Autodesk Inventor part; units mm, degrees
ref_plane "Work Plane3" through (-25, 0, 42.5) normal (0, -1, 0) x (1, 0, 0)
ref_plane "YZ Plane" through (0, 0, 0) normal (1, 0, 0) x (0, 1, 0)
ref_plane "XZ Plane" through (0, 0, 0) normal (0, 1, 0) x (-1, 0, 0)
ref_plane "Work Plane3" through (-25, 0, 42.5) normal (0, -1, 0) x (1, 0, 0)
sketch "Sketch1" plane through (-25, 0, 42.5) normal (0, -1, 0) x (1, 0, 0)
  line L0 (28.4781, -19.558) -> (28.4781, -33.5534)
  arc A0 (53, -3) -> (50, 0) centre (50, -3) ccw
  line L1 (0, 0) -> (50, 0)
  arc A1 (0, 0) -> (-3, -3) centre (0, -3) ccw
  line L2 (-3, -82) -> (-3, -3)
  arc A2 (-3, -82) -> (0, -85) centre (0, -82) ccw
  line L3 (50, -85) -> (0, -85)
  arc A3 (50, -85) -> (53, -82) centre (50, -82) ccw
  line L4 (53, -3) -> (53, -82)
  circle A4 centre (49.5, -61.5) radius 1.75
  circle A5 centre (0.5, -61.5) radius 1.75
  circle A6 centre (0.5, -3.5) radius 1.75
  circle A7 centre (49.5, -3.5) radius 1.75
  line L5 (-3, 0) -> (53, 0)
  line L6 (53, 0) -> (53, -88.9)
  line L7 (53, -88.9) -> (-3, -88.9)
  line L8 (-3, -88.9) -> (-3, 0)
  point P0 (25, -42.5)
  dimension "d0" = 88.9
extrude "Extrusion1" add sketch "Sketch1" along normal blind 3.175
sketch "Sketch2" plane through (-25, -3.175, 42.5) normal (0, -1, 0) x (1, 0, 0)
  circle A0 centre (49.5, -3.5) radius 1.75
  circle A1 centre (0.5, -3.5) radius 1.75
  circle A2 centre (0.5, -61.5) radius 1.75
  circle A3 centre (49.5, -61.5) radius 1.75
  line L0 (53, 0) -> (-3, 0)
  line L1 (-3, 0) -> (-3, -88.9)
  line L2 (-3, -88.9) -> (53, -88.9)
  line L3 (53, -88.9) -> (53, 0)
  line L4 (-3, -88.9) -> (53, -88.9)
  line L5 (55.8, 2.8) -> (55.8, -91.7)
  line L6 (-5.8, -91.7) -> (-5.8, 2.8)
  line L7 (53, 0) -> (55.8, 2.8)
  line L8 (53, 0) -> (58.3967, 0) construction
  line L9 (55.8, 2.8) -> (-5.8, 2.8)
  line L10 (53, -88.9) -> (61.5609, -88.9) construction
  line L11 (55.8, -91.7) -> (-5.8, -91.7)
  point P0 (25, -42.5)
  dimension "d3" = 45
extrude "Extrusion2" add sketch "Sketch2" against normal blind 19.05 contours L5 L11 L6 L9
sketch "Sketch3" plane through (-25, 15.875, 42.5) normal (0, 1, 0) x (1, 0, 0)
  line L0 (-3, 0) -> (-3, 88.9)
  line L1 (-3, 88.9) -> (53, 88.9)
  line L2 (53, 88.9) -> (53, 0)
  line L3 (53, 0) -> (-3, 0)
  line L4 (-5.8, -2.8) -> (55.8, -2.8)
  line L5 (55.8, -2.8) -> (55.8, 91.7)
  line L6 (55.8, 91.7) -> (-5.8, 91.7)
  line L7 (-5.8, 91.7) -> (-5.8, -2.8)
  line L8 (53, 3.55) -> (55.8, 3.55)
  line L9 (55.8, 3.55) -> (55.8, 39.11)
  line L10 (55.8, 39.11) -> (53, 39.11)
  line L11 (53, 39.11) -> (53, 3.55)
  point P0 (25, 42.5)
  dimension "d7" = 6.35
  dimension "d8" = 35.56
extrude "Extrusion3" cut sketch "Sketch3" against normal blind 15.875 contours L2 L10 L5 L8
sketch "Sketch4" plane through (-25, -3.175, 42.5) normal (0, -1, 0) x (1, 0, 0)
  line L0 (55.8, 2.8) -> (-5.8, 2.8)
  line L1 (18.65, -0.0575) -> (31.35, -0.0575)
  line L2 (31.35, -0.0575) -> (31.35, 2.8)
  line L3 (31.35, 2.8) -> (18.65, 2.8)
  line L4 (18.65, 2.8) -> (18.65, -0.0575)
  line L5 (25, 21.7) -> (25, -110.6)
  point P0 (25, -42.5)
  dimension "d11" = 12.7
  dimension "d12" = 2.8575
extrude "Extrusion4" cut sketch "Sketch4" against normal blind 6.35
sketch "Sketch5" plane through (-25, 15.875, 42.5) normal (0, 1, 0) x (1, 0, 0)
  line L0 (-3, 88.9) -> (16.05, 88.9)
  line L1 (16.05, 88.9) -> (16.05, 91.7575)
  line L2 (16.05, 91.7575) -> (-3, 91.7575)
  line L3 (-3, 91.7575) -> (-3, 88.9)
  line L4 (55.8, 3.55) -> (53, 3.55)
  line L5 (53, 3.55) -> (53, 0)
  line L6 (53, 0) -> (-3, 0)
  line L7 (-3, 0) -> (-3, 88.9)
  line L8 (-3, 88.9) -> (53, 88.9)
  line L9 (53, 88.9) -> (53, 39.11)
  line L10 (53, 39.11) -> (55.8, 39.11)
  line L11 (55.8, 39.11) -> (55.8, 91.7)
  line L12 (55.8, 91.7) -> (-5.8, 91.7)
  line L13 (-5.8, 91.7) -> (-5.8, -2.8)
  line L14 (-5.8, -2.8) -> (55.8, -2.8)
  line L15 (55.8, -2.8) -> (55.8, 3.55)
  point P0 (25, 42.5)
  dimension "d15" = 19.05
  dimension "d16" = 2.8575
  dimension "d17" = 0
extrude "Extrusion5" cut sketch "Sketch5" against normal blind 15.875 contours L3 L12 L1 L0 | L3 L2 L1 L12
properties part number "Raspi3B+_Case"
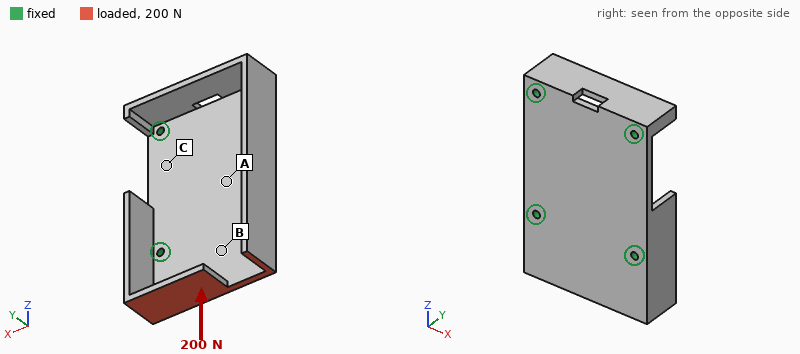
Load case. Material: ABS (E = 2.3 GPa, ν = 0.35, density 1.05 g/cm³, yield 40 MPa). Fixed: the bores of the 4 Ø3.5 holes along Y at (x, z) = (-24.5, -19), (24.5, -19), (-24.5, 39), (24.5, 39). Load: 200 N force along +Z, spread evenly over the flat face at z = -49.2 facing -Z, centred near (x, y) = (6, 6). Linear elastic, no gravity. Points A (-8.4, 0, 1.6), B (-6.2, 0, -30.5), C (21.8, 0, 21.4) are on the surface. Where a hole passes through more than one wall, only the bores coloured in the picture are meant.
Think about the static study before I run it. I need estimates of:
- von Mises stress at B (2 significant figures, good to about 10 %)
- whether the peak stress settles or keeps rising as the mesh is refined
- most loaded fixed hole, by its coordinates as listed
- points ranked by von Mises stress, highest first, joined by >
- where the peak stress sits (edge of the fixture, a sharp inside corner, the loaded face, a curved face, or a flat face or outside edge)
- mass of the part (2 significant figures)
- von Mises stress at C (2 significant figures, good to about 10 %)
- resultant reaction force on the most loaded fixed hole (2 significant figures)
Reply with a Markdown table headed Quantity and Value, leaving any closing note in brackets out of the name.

| Quantity | Value |
|---|---|
| von Mises stress at B | 4.1 MPa |
| whether the peak stress settles or keeps rising as the mesh is refined | keeps rising |
| most loaded fixed hole, by its coordinates as listed | (24.5, -19) |
| points ranked by von Mises stress, highest first, joined by > | B > C > A |
| where the peak stress sits | edge of the fixture |
| mass of the part | 31 g |
| von Mises stress at C | 2.2 MPa |
| resultant reaction force on the most loaded fixed hole | 100 N |
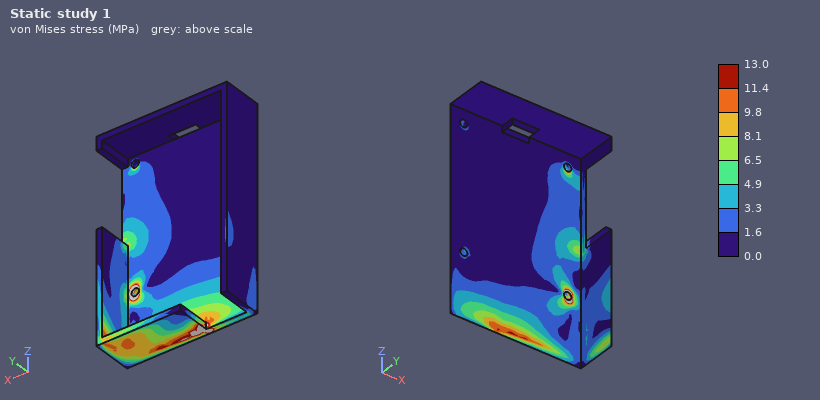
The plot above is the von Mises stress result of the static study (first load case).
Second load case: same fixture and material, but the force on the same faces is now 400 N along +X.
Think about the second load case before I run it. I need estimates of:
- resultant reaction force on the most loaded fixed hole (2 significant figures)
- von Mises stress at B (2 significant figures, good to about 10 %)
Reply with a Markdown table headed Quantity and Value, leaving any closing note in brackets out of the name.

| Quantity | Value |
|---|---|
| resultant reaction force on the most loaded fixed hole | 330 N |
| von Mises stress at B | 9.1 MPa |
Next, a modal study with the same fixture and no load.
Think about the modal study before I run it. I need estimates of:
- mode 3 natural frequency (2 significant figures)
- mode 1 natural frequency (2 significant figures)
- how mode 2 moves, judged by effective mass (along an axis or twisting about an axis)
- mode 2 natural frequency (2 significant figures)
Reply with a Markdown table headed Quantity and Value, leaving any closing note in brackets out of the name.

| Quantity | Value |
|---|---|
| mode 3 natural frequency | 1400 Hz |
| mode 1 natural frequency | 770 Hz |
| how mode 2 moves, judged by effective mass | along Y |
| mode 2 natural frequency | 1100 Hz |
